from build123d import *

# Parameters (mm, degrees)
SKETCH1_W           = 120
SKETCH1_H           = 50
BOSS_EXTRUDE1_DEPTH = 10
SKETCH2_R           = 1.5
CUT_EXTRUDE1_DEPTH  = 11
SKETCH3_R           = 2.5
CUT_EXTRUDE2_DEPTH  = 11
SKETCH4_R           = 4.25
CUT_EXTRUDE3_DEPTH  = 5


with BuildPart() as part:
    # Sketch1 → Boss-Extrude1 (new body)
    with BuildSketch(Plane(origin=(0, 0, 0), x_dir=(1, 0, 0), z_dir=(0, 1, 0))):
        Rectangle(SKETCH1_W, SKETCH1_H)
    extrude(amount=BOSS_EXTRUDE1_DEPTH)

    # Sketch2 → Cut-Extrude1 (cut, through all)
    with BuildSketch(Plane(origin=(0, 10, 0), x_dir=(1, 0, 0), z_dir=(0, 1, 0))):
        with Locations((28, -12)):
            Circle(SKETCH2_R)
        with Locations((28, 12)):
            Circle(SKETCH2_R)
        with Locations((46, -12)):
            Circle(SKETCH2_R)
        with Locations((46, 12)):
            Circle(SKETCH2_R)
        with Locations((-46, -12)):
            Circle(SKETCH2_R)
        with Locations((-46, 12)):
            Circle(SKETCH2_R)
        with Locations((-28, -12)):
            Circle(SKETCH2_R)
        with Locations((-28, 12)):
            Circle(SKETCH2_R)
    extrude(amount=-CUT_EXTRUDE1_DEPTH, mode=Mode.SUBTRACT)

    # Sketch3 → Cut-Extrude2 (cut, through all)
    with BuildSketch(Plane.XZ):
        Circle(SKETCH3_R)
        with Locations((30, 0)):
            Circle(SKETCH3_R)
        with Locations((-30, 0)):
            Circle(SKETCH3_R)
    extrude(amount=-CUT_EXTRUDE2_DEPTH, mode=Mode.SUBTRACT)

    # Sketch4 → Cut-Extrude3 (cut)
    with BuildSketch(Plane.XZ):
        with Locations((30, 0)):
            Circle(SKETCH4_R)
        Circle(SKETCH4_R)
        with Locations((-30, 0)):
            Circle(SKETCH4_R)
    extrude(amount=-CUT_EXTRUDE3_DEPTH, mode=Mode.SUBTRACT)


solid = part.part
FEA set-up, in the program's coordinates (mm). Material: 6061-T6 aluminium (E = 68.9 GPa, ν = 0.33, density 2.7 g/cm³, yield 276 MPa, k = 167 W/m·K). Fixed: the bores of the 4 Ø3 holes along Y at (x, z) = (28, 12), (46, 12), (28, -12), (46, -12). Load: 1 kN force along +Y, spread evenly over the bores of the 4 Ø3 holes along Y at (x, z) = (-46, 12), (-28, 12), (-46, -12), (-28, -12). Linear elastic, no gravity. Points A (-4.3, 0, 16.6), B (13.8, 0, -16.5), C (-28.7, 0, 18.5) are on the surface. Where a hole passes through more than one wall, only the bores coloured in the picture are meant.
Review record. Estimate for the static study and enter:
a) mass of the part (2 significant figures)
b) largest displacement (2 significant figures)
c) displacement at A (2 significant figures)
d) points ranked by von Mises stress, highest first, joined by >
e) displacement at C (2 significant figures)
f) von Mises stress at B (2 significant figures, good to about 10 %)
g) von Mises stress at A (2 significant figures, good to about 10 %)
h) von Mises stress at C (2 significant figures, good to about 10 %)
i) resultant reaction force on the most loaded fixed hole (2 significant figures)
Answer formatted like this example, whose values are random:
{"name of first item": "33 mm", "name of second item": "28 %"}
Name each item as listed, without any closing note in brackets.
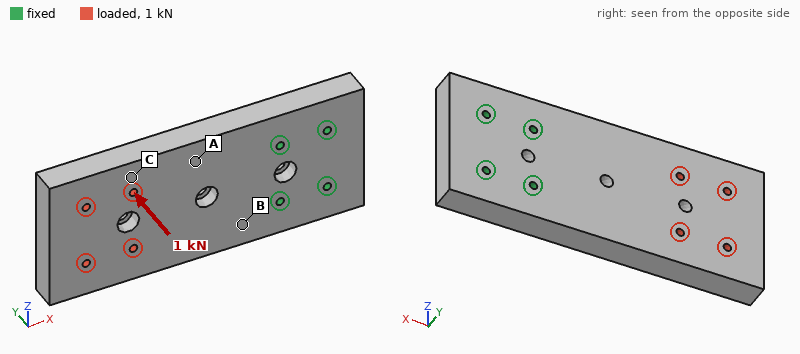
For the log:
{"mass of the part": "160 g", "largest displacement": "0.57 mm", "displacement at A": "0.13 mm", "points ranked by von Mises stress, highest first, joined by >": "B > A > C", "displacement at C": "0.30 mm", "von Mises stress at B": "61 MPa", "von Mises stress at A": "42 MPa", "von Mises stress at C": "13 MPa", "resultant reaction force on the most loaded fixed hole": "1.2 kN"}
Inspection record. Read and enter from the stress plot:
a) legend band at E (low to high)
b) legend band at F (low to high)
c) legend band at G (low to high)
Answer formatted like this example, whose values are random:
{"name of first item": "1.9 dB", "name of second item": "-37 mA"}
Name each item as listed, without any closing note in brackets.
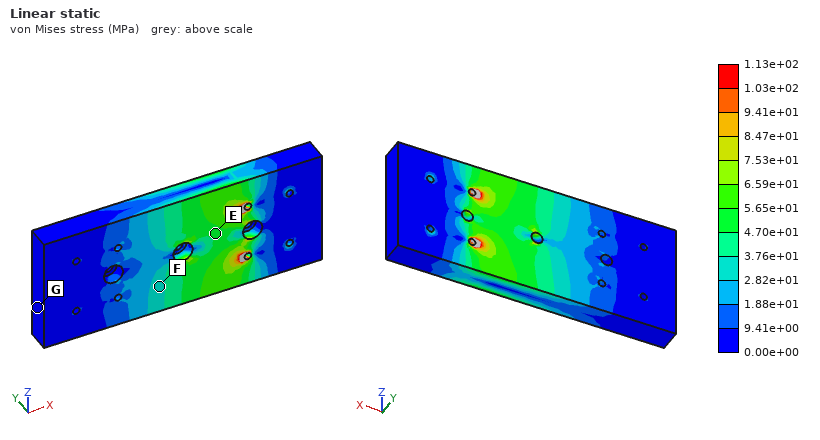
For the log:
{"legend band at E": "4.70e+01 to 5.65e+01 MPa", "legend band at F": "2.82e+01 to 3.76e+01 MPa", "legend band at G": "0.00e+00 to 9.41e+00 MPa"}
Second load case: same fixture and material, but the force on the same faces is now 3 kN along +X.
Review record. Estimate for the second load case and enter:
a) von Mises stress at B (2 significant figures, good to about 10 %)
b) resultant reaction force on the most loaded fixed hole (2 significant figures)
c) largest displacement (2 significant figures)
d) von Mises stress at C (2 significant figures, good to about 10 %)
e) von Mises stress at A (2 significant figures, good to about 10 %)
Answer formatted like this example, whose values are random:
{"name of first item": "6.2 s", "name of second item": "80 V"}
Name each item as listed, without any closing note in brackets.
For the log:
{"von Mises stress at B": "6.9 MPa", "resultant reaction force on the most loaded fixed hole": "1.2 kN", "largest displacement": "7.7 µm", "von Mises stress at C": "4.8 MPa", "von Mises stress at A": "6.6 MPa"}
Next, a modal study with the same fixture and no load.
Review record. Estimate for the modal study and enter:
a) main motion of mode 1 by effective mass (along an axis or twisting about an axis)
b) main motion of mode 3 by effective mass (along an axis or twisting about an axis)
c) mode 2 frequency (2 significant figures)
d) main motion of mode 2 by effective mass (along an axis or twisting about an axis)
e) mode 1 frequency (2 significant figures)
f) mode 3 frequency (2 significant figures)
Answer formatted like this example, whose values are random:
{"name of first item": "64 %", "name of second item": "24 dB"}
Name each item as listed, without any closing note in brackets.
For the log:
{"main motion of mode 1 by effective mass": "along Y", "main motion of mode 3 by effective mass": "along Z", "mode 2 frequency": "3500 Hz", "main motion of mode 2 by effective mass": "twisting about X", "mode 1 frequency": "990 Hz", "mode 3 frequency": "3700 Hz"}
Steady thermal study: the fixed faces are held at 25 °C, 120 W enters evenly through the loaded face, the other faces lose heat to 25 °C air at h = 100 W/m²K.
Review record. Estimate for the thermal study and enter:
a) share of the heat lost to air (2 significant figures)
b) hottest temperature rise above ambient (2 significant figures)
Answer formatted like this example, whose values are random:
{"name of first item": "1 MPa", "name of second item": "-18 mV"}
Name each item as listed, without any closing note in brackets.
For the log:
{"share of the heat lost to air": "41 %", "hottest temperature rise above ambient": "70 K"}
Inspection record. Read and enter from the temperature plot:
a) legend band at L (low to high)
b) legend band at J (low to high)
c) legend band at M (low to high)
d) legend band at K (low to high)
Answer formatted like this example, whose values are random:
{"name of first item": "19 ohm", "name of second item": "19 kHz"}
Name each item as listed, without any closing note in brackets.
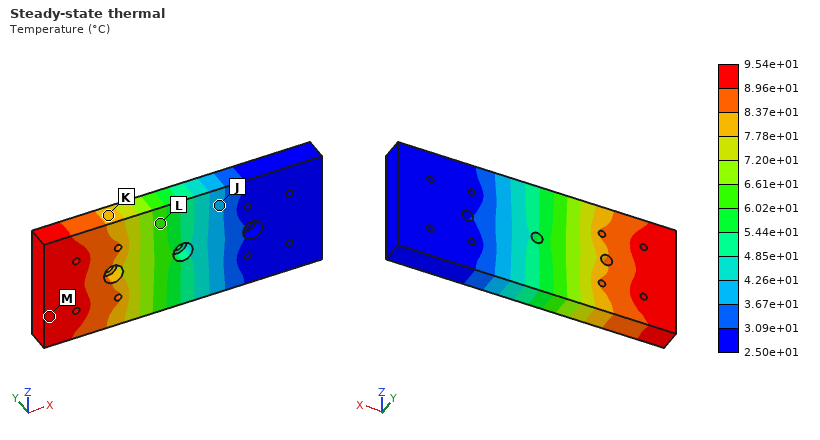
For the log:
{"legend band at L": "6.02e+01 to 6.61e+01 °C", "legend band at J": "3.67e+01 to 4.26e+01 °C", "legend band at M": "8.96e+01 to 9.54e+01 °C", "legend band at K": "7.78e+01 to 8.37e+01 °C"}
